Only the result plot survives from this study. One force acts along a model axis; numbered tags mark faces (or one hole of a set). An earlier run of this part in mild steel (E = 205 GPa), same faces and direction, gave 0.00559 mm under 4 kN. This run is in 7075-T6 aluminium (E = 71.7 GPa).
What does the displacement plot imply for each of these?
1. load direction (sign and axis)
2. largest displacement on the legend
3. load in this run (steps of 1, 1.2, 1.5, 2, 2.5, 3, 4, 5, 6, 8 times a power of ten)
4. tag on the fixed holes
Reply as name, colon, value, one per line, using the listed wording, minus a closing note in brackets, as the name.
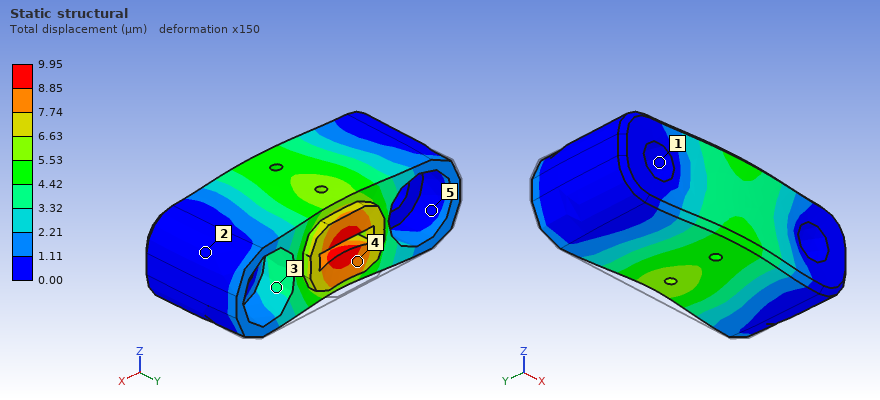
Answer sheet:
load direction: -Y
largest displacement on the legend: 9.95 µm
load in this run: 2.5 kN
tag on the fixed holes: 1
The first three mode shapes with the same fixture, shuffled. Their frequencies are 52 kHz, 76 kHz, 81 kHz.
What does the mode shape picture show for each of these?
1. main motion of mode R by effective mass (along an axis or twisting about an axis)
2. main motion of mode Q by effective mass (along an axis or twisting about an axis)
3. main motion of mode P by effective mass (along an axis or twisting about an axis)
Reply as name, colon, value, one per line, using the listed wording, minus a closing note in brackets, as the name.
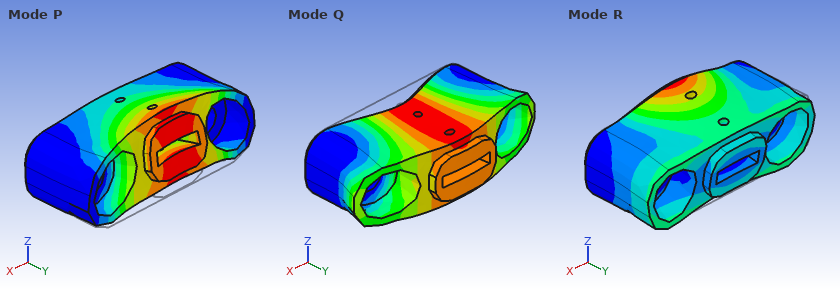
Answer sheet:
main motion of mode R by effective mass: along Z
main motion of mode Q by effective mass: along Y
main motion of mode P by effective mass: along Z
